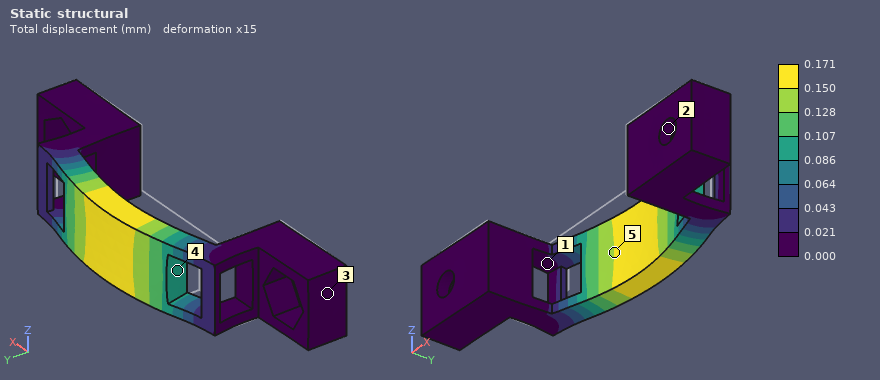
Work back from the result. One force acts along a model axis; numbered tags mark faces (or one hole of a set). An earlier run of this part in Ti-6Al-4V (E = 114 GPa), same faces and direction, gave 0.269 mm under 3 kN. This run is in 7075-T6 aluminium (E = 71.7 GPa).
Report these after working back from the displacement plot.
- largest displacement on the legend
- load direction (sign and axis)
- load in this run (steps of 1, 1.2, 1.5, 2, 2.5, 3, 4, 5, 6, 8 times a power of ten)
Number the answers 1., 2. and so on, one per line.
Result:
1. 0.171 mm
2. +Y
3. 1.2 kN
